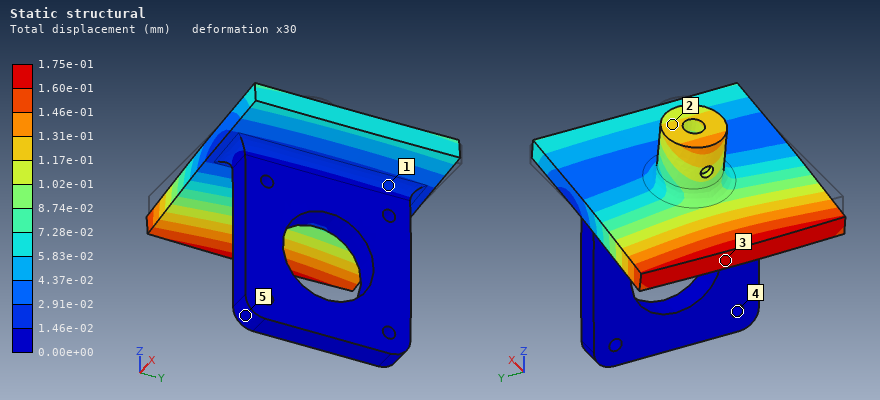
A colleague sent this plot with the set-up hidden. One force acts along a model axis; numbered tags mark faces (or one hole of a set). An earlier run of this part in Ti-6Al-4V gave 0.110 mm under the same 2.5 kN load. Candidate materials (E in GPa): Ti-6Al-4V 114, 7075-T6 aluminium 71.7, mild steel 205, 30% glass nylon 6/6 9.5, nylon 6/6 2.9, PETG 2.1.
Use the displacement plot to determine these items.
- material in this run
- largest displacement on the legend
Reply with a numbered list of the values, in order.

1. 7075-T6 aluminium
2. 1.75e-01 mm
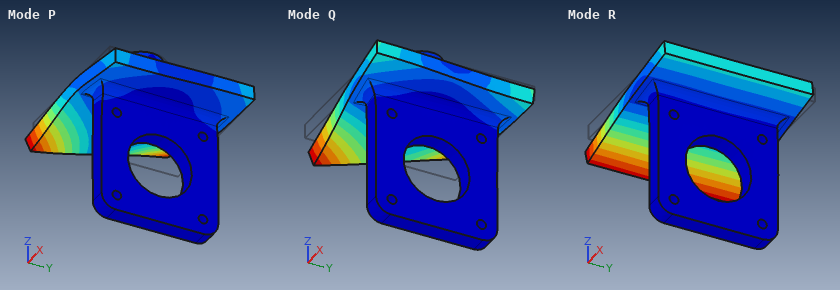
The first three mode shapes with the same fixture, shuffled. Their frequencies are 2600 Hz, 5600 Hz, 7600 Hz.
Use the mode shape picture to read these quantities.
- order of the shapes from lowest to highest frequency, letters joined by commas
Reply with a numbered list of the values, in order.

1. R, Q, P
